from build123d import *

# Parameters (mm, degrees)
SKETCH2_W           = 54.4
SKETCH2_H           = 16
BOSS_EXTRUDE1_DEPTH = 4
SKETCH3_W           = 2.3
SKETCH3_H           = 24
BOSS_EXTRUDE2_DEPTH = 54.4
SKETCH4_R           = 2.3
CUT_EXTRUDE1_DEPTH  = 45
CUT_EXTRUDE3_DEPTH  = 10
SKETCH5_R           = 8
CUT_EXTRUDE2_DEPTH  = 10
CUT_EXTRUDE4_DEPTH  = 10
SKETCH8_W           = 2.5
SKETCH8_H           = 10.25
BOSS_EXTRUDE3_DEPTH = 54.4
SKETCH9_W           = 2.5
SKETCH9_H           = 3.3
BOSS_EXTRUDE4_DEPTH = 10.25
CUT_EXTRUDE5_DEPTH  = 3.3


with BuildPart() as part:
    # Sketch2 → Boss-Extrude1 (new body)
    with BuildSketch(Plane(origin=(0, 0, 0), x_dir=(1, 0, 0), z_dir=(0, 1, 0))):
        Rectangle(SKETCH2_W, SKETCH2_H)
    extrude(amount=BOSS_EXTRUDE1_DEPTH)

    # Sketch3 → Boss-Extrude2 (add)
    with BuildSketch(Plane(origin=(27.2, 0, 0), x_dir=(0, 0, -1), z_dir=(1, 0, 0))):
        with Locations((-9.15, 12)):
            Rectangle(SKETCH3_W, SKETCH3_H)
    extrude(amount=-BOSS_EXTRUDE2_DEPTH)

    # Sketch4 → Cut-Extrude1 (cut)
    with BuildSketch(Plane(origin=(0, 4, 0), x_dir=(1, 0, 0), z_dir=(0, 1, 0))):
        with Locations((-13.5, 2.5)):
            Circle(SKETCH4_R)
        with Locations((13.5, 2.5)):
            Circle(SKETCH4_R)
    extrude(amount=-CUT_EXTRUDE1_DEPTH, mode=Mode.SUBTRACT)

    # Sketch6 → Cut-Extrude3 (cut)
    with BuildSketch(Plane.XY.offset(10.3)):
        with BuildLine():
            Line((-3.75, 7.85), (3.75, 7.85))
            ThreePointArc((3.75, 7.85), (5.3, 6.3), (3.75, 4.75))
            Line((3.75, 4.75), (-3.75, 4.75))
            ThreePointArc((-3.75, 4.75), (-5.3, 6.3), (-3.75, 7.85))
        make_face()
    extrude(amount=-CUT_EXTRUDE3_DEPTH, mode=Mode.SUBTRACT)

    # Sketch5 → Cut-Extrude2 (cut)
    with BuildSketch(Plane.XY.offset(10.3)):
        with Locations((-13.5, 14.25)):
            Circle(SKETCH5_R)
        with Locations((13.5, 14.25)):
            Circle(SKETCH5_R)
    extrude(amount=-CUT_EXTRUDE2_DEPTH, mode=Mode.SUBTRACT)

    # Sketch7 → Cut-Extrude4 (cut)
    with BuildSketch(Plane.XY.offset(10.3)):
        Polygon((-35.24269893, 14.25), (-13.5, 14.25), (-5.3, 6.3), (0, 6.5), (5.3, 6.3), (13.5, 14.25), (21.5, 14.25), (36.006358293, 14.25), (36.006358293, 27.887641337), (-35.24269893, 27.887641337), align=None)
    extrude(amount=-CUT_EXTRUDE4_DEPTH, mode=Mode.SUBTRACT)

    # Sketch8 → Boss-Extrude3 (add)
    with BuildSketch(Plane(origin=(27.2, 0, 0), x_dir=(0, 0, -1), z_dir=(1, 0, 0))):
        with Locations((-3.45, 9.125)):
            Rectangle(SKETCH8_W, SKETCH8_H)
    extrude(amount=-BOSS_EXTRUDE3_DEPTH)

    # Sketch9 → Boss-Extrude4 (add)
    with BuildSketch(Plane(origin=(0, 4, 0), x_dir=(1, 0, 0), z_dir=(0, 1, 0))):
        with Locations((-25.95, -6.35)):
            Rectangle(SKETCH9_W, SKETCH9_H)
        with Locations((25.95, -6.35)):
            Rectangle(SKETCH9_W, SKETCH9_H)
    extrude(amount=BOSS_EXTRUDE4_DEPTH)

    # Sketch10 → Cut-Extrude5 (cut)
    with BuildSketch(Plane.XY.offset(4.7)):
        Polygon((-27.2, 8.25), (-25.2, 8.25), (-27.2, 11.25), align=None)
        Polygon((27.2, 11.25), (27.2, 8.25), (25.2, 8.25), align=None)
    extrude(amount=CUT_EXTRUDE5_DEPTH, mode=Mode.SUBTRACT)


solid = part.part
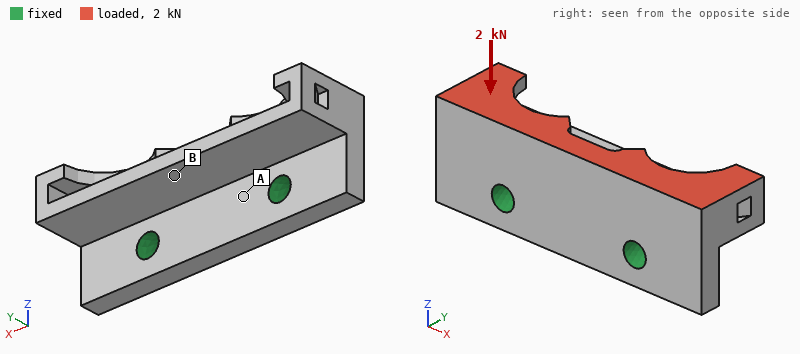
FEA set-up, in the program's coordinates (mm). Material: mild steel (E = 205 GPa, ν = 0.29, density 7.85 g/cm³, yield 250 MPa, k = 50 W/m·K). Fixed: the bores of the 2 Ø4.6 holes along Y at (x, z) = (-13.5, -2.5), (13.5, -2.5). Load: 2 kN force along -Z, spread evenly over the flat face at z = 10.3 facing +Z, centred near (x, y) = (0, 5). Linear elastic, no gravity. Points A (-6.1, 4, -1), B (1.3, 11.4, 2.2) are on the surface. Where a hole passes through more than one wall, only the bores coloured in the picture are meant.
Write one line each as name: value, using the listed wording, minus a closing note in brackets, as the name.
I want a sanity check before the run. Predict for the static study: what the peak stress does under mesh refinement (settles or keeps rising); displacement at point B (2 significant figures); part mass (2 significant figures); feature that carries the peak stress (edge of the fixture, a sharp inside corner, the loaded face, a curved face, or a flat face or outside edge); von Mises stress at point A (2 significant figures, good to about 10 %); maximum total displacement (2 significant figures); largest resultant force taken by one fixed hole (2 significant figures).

what the peak stress does under mesh refinement: keeps rising
displacement at point B: 5.3 µm
part mass: 47 g
feature that carries the peak stress: edge of the fixture
von Mises stress at point A: 20 MPa
maximum total displacement: 21 µm
largest resultant force taken by one fixed hole: 1.0 kN
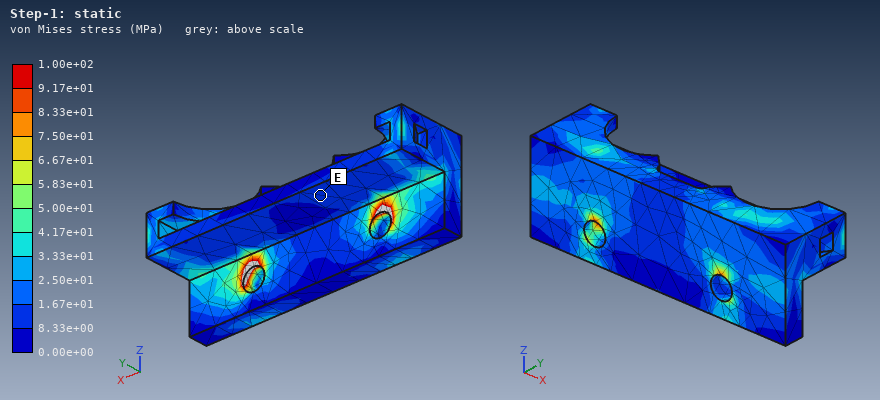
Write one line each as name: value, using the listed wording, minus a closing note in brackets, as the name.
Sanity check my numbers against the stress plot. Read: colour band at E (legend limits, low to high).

colour band at E: 8.33e+00 to 1.67e+01 MPa
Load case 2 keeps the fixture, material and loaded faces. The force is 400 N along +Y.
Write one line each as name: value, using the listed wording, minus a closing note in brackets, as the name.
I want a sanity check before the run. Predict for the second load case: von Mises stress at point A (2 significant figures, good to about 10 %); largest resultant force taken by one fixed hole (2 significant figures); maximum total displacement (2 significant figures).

von Mises stress at point A: 14 MPa
largest resultant force taken by one fixed hole: 200 N
maximum total displacement: 9.4 µm
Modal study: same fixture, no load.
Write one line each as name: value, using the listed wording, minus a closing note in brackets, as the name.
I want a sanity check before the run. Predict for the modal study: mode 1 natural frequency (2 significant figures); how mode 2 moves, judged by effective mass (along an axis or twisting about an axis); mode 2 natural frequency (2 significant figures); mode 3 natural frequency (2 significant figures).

mode 1 natural frequency: 9400 Hz
how mode 2 moves, judged by effective mass: twisting about Z
mode 2 natural frequency: 10 kHz
mode 3 natural frequency: 17 kHz
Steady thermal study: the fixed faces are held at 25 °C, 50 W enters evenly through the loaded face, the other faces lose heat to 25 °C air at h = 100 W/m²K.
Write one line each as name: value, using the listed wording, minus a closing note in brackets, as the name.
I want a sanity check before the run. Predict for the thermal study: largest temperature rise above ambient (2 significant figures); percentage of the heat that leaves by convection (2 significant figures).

largest temperature rise above ambient: 70 K
percentage of the heat that leaves by convection: 24 %
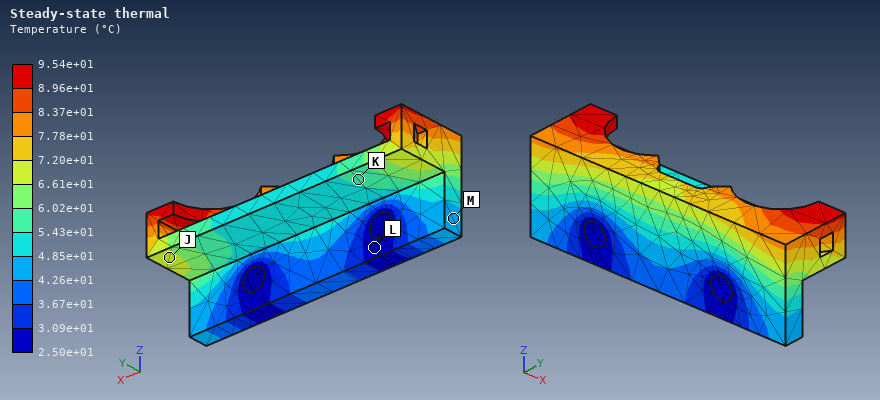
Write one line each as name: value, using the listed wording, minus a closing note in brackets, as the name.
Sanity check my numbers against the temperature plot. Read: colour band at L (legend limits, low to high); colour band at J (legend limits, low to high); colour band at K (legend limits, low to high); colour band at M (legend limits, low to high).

colour band at L: 2.50e+01 to 3.09e+01 °C
colour band at J: 6.61e+01 to 7.20e+01 °C
colour band at K: 5.43e+01 to 6.02e+01 °C
colour band at M: 4.26e+01 to 4.85e+01 °C
